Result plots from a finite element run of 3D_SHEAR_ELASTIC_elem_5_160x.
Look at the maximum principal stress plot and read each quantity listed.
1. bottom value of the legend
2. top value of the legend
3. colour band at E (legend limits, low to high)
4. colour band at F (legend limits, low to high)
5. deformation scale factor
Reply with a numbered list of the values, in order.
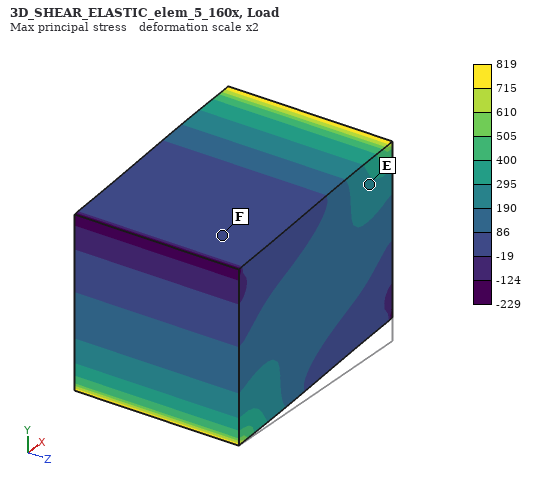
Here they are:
1. -229
2. 819
3. 190 to 295
4. -19 to 86
5. 2
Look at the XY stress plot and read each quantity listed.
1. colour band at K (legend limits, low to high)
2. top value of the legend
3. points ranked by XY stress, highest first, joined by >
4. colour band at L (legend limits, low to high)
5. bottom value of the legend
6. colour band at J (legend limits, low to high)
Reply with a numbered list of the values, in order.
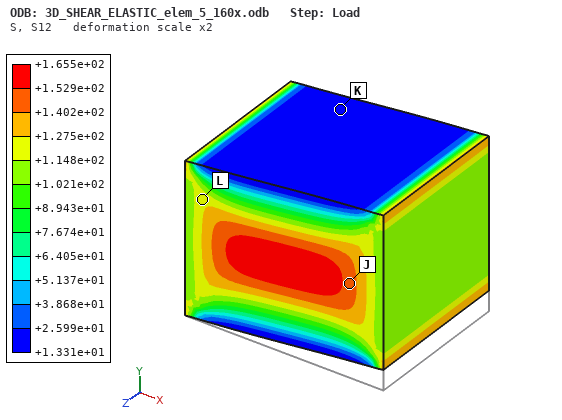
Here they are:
1. +1.331e+01 to +2.599e+01
2. +1.655e+02
3. J > L > K
4. +1.148e+02 to +1.275e+02
5. +1.331e+01
6. +1.402e+02 to +1.529e+02
